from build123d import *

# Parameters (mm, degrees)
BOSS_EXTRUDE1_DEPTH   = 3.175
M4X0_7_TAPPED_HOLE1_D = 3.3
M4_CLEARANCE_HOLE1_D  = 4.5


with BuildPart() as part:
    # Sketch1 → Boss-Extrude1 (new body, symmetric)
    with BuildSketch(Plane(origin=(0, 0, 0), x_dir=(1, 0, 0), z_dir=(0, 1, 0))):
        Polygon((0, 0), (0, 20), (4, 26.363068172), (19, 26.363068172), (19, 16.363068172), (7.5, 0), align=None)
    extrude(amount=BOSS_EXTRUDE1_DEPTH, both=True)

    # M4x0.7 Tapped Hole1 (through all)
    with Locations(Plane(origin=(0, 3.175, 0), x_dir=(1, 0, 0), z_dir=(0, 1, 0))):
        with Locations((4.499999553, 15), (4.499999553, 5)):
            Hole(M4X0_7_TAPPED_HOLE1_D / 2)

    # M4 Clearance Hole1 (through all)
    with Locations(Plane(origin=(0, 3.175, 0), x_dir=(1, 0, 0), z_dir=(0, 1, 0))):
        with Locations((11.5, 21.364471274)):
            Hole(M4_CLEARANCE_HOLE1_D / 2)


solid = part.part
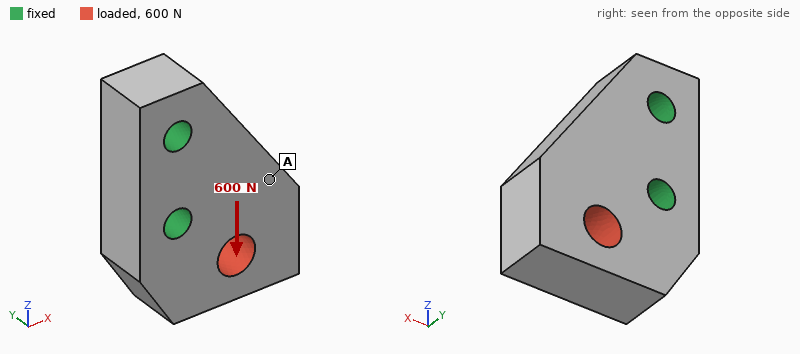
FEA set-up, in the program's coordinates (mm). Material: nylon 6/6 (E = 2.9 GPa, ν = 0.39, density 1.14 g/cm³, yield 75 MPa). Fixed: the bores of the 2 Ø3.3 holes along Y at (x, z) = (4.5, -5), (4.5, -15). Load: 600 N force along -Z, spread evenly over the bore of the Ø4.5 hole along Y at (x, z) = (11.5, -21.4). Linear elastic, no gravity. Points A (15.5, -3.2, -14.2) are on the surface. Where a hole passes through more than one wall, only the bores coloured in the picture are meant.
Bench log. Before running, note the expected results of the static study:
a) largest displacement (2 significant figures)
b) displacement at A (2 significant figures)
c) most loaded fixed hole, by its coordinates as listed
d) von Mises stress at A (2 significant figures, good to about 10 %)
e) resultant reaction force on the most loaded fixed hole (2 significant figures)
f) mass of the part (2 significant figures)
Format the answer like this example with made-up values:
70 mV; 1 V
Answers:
0.12 mm; 0.073 mm; (4.5, -15); 7.6 MPa; 470 N; 2.6 g
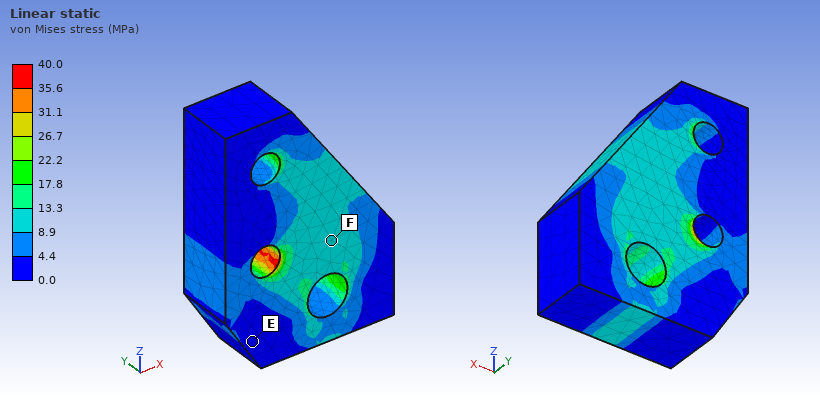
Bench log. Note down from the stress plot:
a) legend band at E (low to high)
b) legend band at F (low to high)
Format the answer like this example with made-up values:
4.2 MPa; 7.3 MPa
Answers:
0.0 to 4.4 MPa; 8.9 to 13.3 MPa
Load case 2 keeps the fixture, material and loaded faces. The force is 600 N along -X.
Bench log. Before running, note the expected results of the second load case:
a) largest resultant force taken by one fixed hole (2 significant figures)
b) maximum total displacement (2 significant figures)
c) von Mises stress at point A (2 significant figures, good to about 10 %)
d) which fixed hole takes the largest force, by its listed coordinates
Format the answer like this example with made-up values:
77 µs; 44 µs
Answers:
830 N; 0.18 mm; 6.0 MPa; (4.5, -15)
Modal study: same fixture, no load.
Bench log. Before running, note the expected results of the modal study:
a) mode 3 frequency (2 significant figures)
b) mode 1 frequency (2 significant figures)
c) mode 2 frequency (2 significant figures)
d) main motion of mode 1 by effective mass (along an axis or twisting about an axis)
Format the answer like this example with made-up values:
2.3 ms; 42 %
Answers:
12 kHz; 6200 Hz; 9200 Hz; along Y
